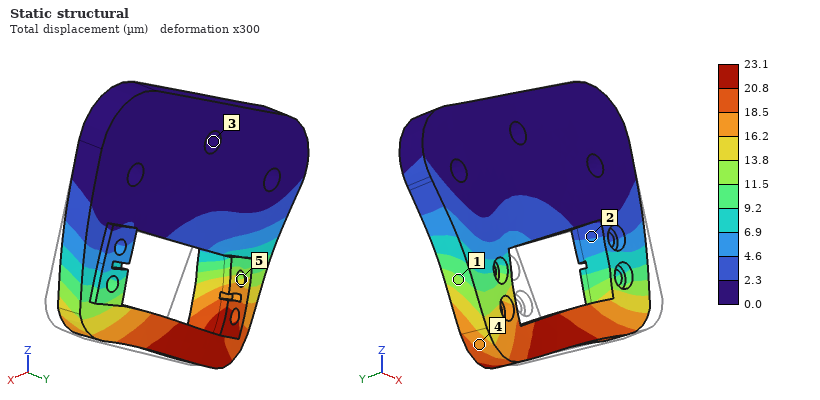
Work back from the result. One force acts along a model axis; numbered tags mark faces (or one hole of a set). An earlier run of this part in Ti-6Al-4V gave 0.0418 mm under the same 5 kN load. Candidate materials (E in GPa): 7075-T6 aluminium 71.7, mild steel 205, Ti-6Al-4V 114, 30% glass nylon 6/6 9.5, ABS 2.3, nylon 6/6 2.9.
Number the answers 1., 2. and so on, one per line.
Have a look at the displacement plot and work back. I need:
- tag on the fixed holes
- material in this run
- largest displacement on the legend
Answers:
1. 3
2. mild steel
3. 23.1 µm
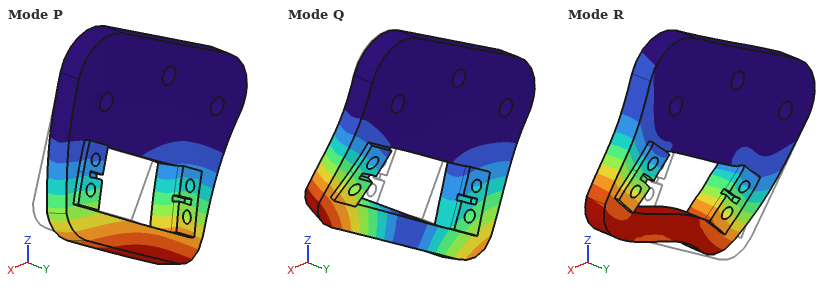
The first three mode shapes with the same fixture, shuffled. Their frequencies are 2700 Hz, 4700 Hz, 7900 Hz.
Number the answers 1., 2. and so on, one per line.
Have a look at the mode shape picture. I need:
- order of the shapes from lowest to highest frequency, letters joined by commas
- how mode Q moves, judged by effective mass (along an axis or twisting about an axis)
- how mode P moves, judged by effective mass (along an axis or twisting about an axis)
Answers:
1. P, Q, R
2. twisting about Z
3. along Y
